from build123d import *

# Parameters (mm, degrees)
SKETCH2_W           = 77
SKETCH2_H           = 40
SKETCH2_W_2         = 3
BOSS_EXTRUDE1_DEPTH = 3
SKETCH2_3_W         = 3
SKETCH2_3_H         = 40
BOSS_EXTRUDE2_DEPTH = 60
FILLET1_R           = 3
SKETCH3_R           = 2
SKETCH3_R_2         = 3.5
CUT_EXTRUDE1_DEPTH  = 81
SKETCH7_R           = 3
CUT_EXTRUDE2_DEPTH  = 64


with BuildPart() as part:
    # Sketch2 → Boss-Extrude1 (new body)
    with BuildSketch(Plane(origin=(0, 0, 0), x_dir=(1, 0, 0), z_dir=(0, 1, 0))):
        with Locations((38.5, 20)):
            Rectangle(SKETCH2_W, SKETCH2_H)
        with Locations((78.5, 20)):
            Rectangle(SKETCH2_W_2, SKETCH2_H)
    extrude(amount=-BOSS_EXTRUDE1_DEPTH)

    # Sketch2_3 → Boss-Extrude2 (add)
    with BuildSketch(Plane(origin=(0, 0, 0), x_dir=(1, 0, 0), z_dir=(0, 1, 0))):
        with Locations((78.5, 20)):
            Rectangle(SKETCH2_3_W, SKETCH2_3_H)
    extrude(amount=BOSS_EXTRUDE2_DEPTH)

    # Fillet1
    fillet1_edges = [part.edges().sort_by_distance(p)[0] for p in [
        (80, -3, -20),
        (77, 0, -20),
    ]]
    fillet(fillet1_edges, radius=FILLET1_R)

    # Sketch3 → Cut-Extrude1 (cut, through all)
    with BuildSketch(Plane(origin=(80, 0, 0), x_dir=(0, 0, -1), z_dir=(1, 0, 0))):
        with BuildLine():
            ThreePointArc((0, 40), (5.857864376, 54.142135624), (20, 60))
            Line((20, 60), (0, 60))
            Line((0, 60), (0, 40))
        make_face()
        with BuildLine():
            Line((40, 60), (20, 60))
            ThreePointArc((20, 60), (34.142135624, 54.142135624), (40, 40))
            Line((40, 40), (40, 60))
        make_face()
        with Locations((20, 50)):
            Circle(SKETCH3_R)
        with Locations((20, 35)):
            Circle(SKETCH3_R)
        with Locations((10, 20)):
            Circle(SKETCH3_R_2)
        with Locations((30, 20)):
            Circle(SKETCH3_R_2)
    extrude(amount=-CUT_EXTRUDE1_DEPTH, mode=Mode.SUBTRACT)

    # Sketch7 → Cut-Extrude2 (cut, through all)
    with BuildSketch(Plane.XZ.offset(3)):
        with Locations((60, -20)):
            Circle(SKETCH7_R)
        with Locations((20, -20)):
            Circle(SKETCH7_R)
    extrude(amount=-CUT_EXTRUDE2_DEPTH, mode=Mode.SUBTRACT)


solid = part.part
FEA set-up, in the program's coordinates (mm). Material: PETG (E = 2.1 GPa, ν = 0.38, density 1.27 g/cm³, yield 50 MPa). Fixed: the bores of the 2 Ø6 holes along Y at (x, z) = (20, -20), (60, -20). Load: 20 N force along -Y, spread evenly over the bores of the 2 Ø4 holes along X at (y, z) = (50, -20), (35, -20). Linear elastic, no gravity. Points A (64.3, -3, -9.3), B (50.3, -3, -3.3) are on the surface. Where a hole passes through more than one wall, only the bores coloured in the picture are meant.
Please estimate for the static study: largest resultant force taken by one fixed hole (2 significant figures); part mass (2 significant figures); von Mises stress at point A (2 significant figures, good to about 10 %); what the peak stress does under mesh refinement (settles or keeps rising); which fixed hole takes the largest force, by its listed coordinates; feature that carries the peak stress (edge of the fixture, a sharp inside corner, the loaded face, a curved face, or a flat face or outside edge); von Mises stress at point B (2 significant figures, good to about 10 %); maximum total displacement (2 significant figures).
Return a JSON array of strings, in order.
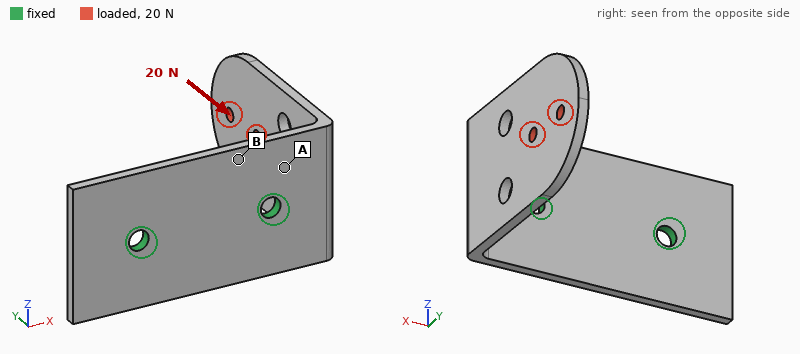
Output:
["22 N", "20 g", "3.1 MPa", "keeps rising", "(60, -20)", "edge of the fixture", "0.82 MPa", "1.1 mm"]
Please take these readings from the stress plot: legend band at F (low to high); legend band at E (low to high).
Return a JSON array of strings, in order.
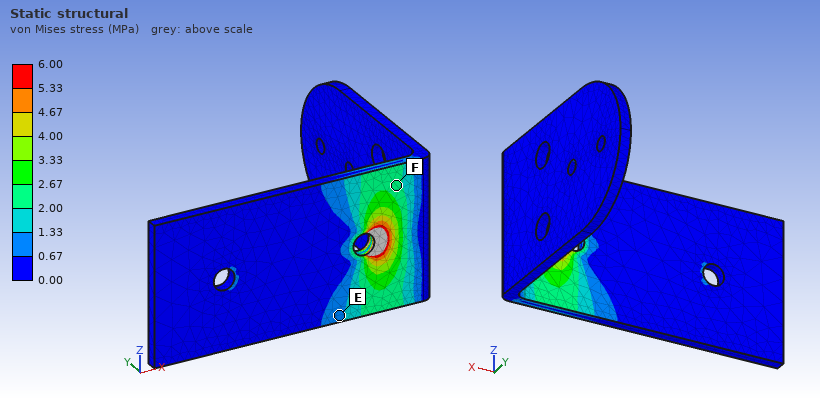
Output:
["2.00 to 2.67 MPa", "0.67 to 1.33 MPa"]
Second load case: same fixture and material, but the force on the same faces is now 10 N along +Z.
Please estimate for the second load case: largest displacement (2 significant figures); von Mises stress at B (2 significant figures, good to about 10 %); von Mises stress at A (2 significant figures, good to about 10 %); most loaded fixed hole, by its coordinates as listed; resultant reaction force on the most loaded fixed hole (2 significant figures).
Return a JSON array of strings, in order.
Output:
["1.3 mm", "2.2 MPa", "2.9 MPa", "(60, -20)", "14 N"]
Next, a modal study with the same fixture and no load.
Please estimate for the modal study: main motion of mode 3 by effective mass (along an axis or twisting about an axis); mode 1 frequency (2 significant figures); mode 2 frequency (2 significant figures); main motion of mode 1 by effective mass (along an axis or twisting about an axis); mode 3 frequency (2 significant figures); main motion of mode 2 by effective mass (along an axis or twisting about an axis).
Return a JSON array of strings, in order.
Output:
["along Y", "130 Hz", "220 Hz", "along X", "600 Hz", "along Z"]
